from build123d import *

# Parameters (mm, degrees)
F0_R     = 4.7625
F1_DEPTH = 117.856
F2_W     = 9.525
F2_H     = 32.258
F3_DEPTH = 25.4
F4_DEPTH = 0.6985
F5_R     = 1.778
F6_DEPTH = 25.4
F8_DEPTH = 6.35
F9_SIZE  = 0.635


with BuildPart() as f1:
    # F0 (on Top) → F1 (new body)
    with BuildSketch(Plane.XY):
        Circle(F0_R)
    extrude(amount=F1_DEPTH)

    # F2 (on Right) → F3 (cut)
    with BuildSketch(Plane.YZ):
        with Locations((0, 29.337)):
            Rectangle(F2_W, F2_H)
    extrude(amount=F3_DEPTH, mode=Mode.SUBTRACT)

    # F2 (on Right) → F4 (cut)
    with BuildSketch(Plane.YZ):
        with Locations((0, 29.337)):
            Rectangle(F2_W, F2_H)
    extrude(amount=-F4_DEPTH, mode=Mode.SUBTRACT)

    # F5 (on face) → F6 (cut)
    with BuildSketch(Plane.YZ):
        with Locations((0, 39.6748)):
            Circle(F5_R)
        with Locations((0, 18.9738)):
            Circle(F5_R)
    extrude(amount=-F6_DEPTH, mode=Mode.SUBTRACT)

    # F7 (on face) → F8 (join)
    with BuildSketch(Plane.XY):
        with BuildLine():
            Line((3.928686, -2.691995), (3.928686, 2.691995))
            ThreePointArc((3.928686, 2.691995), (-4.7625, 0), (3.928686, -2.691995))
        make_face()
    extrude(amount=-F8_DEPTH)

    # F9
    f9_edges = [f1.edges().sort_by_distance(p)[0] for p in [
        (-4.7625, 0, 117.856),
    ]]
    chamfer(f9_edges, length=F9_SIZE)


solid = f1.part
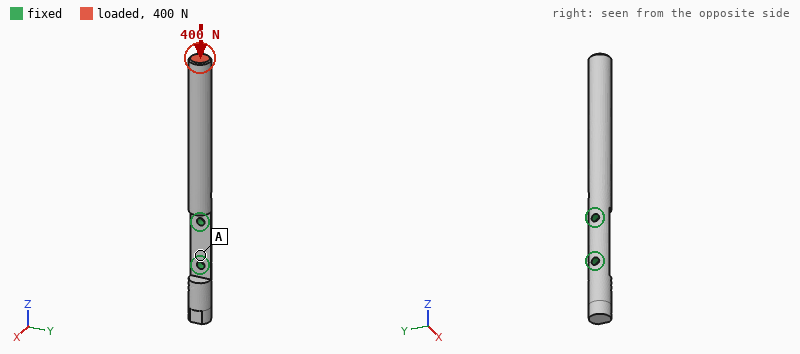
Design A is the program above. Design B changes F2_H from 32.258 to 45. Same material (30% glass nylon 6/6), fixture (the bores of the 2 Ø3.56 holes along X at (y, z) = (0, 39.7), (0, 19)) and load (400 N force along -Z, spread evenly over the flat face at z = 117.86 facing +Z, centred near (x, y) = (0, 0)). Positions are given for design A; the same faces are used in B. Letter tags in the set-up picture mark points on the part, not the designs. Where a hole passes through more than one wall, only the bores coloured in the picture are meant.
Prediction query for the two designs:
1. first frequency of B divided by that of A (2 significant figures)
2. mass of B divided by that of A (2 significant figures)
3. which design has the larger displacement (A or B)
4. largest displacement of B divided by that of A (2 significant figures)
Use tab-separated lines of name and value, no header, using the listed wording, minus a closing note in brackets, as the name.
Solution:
first frequency of B divided by that of A	0.79
mass of B divided by that of A	0.93
which design has the larger displacement	B
largest displacement of B divided by that of A	1.9
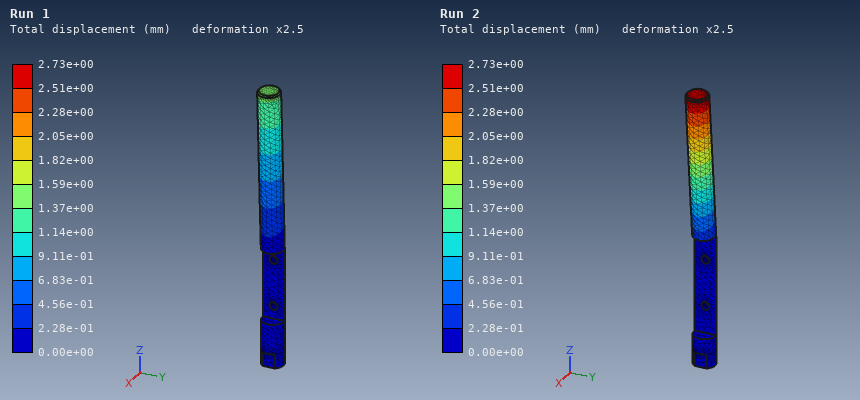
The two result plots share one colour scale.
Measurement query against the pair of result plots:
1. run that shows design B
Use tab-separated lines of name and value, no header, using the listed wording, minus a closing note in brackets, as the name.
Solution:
run that shows design B	Run 2
